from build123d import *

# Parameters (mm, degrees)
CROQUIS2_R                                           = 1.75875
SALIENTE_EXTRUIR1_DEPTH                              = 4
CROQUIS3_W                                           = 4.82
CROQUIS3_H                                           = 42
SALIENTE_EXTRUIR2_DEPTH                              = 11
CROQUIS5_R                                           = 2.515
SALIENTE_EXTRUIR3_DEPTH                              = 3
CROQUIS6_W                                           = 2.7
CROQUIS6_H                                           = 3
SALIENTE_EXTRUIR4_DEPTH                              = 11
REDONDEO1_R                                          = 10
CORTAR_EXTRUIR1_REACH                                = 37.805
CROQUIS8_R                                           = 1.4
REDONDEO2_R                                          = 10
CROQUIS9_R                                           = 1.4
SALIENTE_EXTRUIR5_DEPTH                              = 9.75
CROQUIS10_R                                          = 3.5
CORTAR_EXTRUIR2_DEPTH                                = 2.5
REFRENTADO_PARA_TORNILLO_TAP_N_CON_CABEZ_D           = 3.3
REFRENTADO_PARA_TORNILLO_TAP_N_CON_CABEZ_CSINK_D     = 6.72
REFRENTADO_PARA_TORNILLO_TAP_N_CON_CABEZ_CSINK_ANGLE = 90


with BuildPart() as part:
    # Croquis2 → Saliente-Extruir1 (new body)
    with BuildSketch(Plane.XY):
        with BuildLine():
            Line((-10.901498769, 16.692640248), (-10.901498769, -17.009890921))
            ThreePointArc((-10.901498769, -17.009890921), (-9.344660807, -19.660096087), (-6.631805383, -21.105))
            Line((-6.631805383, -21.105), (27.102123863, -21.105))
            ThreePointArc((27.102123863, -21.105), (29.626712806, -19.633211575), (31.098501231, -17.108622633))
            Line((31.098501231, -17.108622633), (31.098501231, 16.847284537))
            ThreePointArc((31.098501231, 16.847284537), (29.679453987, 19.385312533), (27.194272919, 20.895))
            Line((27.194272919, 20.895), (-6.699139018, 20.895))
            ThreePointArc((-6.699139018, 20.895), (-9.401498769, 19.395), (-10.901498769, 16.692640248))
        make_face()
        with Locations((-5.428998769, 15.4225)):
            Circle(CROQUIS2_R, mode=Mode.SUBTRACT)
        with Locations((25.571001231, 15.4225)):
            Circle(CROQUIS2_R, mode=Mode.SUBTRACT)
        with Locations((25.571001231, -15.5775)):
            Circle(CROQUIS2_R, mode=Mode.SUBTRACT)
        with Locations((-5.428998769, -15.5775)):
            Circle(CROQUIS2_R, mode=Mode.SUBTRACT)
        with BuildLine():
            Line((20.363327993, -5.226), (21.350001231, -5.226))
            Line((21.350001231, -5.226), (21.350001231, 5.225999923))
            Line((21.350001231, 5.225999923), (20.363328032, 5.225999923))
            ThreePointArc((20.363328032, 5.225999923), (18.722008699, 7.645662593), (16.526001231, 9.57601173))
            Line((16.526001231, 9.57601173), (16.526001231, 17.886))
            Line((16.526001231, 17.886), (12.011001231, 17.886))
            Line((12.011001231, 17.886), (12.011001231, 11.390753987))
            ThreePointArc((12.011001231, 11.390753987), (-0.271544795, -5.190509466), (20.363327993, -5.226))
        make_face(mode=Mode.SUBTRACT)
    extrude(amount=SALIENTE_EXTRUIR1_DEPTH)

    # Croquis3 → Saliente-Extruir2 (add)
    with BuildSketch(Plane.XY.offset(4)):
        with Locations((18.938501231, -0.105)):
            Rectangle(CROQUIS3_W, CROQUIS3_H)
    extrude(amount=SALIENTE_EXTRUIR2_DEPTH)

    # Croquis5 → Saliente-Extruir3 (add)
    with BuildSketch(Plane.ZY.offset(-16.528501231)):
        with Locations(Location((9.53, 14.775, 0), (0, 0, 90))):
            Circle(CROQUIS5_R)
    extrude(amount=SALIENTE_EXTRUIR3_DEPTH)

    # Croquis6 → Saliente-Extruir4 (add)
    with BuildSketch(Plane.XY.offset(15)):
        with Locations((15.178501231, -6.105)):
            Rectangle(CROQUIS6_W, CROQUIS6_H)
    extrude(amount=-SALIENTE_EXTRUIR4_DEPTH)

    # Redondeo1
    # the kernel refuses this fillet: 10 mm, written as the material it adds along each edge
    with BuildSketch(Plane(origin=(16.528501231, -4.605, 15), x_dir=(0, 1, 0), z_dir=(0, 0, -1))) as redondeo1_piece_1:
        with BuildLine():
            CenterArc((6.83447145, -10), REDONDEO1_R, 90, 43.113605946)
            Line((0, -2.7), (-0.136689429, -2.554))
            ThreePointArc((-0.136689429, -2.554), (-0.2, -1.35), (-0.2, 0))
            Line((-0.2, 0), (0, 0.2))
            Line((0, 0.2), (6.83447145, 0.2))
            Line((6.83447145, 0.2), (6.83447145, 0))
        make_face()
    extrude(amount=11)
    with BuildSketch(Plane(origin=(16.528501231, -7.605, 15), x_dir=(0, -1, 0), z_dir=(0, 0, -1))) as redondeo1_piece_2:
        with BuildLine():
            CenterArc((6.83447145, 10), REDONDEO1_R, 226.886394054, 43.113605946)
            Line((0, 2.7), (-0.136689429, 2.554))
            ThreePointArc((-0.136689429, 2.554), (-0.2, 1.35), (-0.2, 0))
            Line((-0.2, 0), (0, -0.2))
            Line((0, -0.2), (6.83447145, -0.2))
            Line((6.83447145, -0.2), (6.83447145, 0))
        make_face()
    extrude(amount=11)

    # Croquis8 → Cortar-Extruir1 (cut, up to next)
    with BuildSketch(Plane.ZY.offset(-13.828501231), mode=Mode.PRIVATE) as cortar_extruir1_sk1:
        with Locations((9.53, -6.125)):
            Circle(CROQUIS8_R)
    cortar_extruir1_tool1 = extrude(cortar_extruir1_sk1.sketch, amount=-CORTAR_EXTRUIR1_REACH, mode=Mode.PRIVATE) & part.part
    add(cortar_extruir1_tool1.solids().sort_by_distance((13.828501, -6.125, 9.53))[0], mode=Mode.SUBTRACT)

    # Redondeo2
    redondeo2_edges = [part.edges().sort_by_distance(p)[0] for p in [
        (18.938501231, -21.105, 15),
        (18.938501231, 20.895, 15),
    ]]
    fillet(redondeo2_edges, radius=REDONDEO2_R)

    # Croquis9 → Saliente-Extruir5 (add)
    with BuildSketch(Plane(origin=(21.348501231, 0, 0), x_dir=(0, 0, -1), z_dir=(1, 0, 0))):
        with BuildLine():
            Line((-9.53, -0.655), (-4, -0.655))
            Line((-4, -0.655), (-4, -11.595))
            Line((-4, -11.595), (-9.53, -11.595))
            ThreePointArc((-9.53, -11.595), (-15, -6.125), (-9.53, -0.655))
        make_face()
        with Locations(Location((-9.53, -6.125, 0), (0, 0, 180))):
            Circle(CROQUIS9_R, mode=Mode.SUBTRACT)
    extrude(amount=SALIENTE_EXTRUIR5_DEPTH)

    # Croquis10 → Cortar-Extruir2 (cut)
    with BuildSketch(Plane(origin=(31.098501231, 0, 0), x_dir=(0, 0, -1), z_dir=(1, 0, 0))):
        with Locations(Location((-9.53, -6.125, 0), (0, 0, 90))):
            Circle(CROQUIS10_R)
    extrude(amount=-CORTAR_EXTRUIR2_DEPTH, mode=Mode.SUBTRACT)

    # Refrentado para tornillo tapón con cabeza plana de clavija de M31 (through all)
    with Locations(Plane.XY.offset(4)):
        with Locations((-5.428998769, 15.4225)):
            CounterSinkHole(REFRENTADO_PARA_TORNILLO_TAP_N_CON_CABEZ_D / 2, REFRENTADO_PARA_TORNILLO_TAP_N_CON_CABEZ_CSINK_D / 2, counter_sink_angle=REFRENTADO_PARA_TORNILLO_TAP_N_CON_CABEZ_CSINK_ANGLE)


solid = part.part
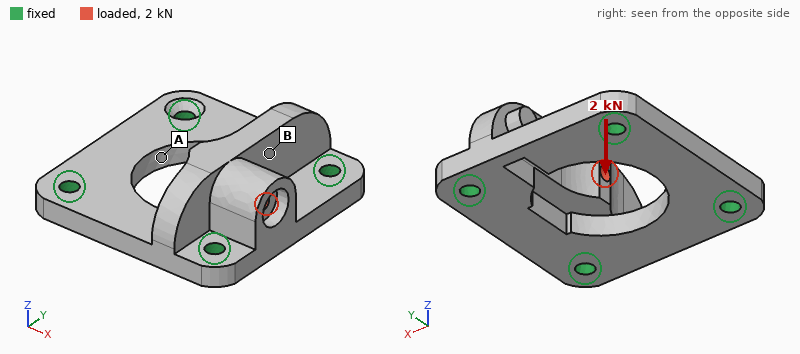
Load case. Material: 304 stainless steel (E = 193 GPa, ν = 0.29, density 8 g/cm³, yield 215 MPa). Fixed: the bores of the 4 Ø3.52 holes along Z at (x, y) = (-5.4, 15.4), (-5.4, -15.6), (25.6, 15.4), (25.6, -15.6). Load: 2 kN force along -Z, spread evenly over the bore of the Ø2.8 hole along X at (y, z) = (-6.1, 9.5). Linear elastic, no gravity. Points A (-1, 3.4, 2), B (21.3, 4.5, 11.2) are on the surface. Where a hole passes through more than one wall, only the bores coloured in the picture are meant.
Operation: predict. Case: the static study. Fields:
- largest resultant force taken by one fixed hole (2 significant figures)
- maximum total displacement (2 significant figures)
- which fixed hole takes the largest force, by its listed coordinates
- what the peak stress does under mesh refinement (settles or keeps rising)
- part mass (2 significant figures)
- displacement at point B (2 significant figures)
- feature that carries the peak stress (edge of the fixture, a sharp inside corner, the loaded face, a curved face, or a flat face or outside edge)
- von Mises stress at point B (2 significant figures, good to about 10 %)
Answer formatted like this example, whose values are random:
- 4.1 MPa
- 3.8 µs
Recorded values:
- 1.4 kN
- 12 µm
- (25.6, -15.6)
- keeps rising
- 65 g
- 7.0 µm
- a sharp inside corner
- 24 MPa
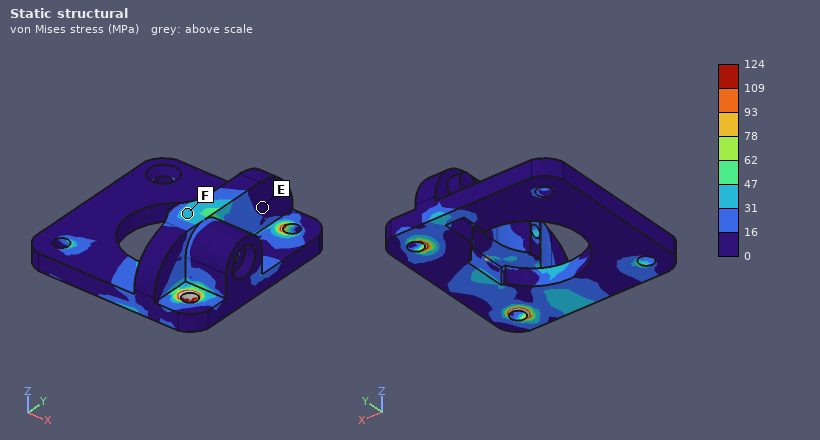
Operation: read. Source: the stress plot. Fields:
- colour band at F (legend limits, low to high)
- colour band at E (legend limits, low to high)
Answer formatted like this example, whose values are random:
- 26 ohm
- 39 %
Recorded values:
- 31 to 47 MPa
- 0 to 16 MPa
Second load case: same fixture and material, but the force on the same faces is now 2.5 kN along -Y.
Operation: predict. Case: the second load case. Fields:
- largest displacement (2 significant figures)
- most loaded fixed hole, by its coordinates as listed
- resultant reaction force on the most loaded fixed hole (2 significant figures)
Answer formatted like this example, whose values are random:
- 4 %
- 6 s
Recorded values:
- 6.2 µm
- (25.6, -15.6)
- 1.5 kN
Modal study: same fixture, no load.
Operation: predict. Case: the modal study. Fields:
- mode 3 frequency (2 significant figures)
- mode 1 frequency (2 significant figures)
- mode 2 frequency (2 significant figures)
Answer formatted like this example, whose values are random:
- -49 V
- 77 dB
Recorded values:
- 19 kHz
- 10 kHz
- 17 kHz
